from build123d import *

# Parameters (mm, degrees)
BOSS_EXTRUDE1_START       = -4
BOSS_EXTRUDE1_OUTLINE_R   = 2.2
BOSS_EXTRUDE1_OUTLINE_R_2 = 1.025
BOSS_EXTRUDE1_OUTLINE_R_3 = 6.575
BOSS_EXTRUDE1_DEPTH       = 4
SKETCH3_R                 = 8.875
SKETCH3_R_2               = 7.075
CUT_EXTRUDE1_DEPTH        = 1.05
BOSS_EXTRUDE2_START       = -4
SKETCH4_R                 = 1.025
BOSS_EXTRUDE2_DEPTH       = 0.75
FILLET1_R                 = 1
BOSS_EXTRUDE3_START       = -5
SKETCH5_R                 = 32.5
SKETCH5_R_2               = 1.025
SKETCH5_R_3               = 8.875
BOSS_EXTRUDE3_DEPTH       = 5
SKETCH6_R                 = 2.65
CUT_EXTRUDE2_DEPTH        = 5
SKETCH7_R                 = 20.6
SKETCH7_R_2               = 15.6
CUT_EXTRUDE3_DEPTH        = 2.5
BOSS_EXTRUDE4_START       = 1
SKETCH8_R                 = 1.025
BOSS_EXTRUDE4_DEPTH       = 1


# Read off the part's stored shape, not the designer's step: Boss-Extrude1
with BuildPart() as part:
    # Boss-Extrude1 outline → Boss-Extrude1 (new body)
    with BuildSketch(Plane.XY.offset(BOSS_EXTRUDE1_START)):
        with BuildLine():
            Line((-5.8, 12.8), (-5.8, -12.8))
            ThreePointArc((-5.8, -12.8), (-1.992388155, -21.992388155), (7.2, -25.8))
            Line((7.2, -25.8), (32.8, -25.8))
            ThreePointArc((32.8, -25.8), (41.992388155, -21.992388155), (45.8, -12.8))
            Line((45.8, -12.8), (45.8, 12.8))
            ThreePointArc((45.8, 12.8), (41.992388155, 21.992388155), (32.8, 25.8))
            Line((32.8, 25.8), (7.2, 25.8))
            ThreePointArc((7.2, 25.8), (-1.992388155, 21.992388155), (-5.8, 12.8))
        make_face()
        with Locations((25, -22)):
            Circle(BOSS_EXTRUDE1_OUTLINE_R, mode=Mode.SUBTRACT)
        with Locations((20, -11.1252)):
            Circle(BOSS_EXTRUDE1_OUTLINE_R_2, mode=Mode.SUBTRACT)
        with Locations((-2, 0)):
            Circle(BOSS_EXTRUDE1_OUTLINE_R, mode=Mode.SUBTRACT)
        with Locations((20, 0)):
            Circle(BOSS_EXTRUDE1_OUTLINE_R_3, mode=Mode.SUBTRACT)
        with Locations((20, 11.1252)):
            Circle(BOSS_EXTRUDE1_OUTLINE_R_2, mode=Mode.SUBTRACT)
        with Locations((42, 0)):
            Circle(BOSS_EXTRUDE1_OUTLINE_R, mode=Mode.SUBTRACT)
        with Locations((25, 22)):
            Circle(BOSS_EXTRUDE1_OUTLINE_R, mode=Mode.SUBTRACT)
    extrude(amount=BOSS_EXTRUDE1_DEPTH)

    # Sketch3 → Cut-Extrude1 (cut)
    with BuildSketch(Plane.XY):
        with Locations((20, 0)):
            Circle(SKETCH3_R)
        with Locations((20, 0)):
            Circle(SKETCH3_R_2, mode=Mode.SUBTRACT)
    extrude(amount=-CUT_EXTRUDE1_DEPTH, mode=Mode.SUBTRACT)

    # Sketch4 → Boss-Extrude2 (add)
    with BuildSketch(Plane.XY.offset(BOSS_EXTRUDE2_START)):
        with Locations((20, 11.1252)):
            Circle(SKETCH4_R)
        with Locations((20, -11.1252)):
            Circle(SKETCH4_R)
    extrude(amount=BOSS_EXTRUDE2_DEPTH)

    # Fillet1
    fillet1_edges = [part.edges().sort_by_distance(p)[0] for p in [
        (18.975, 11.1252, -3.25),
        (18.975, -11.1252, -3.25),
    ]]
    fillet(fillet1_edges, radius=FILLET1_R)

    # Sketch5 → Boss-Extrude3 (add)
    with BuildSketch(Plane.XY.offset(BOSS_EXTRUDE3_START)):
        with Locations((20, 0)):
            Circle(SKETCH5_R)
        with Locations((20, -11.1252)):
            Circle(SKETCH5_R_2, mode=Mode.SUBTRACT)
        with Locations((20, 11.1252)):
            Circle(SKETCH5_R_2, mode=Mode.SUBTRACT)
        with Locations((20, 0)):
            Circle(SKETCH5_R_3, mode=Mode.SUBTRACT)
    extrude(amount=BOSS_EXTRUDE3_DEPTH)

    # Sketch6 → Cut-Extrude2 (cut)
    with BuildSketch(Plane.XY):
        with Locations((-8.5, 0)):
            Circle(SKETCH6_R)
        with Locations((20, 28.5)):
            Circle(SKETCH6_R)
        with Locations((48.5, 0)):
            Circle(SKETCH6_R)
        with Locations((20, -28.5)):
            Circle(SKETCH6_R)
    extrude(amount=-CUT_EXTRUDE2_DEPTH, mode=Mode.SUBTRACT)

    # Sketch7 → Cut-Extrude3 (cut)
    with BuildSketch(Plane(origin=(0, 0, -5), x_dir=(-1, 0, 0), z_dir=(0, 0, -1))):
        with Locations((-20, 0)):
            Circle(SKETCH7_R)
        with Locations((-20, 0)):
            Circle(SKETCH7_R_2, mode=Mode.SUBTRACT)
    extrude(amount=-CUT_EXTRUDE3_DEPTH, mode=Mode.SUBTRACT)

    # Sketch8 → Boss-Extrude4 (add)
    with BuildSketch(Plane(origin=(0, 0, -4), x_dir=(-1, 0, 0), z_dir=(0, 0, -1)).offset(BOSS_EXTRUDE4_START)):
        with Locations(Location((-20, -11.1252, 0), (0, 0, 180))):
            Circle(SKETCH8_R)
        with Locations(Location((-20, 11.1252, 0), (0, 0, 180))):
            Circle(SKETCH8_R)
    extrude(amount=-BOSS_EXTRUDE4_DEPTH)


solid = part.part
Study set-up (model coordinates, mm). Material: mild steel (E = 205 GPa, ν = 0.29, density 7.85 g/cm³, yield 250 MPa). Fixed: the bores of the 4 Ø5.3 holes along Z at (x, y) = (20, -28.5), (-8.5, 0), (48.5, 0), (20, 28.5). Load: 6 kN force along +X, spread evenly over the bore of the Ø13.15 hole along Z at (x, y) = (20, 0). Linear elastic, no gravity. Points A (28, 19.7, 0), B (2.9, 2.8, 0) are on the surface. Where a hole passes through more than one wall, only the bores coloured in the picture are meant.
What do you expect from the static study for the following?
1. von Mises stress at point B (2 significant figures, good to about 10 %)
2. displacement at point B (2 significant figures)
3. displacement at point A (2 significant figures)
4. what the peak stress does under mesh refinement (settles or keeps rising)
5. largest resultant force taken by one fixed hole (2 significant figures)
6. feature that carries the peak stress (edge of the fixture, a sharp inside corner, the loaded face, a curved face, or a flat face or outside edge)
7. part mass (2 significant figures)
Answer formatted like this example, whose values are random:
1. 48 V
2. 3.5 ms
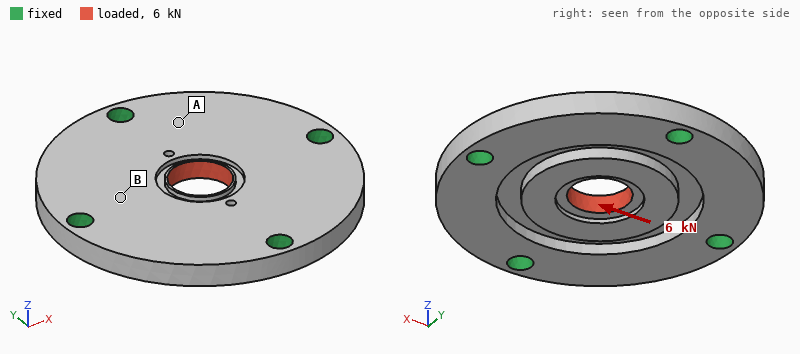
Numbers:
1. 28 MPa
2. 3.0 µm
3. 1.6 µm
4. keeps rising
5. 1.8 kN
6. a sharp inside corner
7. 110 g
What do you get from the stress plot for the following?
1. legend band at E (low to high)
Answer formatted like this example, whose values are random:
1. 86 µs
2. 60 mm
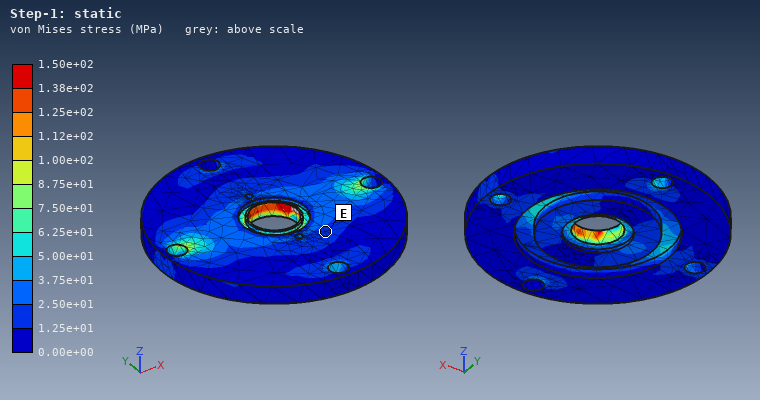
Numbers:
1. 1.25e+01 to 2.50e+01 MPa
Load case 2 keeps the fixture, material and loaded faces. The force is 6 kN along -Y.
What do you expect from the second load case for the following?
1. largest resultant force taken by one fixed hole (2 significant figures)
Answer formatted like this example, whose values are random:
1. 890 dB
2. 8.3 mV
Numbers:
1. 1.8 kN
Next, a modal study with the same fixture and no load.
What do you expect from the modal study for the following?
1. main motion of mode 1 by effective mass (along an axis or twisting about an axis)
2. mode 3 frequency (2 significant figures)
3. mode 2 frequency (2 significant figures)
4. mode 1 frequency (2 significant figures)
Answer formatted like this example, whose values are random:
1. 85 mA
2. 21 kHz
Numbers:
1. along Z
2. 14 kHz
3. 14 kHz
4. 11 kHz
